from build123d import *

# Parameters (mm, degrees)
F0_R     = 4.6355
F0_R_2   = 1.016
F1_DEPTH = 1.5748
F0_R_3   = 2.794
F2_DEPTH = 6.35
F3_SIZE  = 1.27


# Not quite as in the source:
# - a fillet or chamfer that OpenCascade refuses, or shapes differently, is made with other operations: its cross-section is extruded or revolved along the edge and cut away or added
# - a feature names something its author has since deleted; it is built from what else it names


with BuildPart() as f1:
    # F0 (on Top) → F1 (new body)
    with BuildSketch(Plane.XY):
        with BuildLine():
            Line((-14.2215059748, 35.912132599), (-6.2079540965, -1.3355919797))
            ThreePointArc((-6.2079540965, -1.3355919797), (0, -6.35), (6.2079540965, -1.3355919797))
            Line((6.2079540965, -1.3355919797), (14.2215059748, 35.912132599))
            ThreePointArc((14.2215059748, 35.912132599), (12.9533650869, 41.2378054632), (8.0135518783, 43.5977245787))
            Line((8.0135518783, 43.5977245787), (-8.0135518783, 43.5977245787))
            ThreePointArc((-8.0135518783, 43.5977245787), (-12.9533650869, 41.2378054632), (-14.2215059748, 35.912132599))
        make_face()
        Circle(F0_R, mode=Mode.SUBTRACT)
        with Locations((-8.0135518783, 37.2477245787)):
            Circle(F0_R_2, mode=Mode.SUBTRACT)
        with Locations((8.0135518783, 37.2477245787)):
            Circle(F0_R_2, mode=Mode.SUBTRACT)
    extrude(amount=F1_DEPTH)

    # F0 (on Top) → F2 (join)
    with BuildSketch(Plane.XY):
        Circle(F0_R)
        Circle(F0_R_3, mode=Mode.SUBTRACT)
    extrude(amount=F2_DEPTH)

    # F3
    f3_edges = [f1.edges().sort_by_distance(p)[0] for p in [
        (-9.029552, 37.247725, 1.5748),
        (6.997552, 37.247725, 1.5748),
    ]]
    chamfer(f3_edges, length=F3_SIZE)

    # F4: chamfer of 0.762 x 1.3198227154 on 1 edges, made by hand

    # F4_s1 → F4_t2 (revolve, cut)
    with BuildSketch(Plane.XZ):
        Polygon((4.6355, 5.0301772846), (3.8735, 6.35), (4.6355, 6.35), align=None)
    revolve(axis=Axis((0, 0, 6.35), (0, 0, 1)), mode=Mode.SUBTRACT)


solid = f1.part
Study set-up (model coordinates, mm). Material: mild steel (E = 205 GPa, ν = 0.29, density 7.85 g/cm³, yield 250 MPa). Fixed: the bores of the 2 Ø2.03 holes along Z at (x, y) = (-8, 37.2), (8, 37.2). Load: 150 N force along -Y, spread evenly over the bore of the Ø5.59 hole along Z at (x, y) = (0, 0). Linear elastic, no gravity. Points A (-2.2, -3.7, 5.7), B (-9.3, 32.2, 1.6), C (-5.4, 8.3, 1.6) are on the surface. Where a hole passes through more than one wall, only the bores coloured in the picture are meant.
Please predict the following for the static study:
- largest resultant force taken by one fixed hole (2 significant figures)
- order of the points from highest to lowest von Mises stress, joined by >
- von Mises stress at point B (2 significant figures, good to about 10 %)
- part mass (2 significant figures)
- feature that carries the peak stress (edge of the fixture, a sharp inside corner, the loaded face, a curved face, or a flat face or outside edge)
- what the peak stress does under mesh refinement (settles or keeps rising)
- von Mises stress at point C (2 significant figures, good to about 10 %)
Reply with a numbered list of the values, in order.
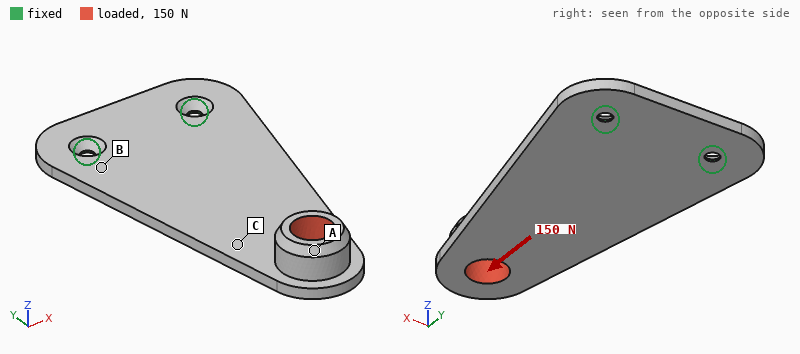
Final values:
1. 76 N
2. C > B > A
3. 34 MPa
4. 14 g
5. edge of the fixture
6. keeps rising
7. 56 MPa
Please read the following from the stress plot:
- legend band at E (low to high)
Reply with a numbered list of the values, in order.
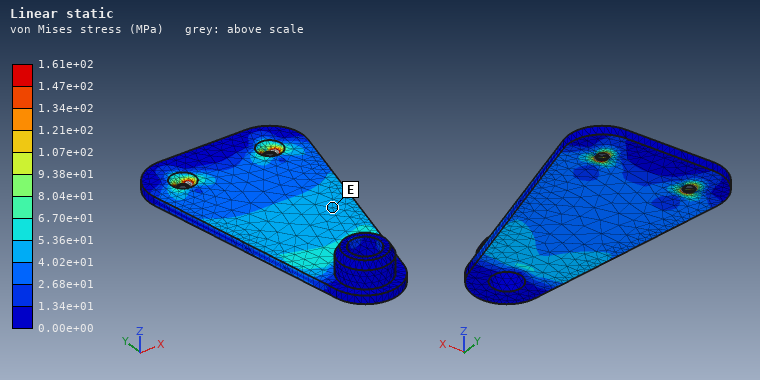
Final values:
1. 4.02e+01 to 5.36e+01 MPa
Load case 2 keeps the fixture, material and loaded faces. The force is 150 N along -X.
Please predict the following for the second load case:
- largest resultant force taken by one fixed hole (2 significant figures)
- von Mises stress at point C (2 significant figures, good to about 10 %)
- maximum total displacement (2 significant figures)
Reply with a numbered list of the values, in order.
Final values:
1. 350 N
2. 49 MPa
3. 44 µm
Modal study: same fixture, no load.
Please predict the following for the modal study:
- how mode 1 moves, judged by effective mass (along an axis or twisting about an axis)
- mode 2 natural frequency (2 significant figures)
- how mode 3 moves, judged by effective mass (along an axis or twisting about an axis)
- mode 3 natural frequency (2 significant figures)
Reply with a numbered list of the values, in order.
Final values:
1. along Z
2. 3600 Hz
3. twisting about Y
4. 4000 Hz
